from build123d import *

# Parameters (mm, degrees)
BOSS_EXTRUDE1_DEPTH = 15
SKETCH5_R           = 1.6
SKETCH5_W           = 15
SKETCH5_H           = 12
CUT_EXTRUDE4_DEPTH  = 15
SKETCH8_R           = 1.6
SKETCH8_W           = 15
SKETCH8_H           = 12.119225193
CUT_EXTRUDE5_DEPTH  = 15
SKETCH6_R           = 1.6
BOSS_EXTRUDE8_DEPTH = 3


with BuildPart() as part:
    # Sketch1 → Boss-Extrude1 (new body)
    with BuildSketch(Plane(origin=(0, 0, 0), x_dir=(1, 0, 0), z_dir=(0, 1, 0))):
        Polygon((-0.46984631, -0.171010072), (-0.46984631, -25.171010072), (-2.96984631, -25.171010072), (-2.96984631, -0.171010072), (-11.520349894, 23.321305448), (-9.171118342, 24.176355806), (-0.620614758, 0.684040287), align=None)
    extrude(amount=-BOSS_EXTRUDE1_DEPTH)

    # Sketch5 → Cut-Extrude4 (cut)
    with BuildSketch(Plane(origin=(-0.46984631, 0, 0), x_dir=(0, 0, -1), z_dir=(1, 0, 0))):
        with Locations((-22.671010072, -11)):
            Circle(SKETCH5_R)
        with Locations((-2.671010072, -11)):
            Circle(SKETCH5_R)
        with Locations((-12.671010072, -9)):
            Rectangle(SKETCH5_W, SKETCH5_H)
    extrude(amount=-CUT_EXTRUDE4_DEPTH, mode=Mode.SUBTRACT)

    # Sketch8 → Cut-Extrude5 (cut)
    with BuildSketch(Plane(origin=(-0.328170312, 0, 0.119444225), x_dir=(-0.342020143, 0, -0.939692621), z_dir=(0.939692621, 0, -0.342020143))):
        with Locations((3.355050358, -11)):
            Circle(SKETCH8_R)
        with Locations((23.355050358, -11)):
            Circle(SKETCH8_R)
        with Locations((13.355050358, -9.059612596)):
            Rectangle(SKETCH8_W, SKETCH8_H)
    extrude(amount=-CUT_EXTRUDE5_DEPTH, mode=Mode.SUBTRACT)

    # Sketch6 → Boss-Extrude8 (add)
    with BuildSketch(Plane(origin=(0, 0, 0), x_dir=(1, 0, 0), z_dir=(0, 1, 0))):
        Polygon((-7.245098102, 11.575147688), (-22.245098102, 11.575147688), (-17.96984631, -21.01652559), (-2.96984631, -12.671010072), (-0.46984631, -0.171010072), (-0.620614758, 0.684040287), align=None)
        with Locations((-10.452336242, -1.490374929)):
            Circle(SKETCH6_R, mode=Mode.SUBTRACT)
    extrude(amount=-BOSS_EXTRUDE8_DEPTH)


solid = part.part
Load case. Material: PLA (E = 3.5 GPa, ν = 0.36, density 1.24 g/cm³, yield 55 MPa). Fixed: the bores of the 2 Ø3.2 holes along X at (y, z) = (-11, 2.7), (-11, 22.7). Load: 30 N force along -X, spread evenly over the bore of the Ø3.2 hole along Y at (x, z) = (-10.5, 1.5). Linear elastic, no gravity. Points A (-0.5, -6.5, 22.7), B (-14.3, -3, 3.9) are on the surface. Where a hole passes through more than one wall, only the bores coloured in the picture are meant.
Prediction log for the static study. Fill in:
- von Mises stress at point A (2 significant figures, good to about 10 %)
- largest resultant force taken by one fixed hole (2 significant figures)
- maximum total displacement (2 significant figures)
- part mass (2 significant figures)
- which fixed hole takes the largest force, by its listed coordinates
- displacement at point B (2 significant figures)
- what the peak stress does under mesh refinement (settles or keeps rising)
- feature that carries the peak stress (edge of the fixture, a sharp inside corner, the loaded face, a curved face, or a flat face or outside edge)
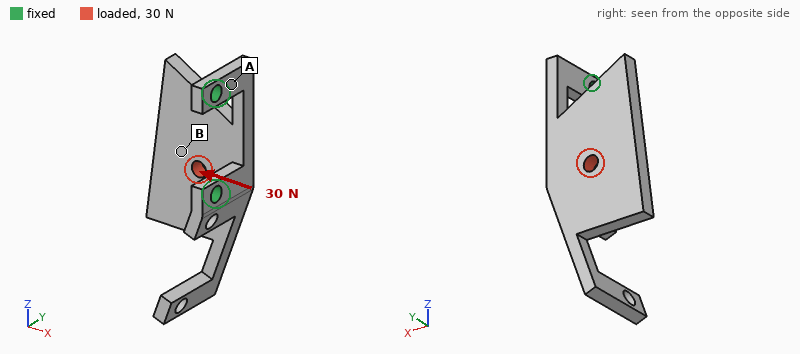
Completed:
4.7 MPa
28 N
0.51 mm
2.9 g
(-11, 2.7)
0.30 mm
keeps rising
edge of the fixture
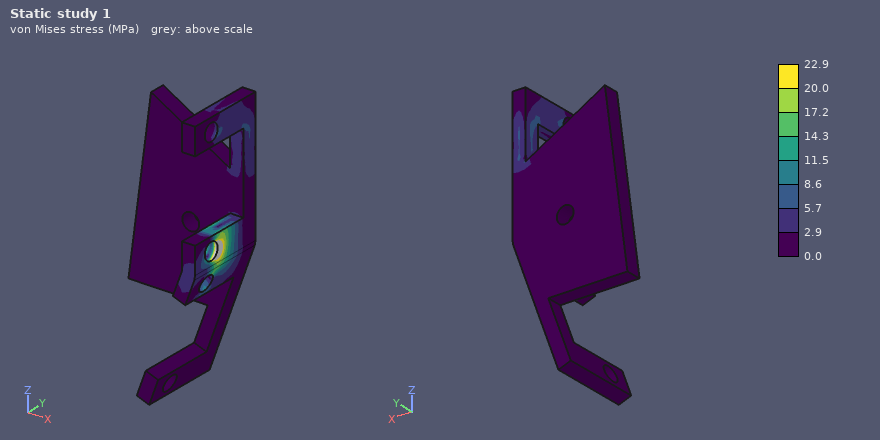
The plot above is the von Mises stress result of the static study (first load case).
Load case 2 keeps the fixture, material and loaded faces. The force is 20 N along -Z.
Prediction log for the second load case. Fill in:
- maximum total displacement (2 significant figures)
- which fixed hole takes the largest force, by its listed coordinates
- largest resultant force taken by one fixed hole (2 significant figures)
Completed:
0.29 mm
(-11, 2.7)
14 N
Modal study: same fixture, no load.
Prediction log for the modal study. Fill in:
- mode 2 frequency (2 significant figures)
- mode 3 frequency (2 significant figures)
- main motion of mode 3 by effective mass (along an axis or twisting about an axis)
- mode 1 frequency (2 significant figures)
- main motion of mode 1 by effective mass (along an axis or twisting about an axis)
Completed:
890 Hz
1100 Hz
twisting about X
680 Hz
along Y
